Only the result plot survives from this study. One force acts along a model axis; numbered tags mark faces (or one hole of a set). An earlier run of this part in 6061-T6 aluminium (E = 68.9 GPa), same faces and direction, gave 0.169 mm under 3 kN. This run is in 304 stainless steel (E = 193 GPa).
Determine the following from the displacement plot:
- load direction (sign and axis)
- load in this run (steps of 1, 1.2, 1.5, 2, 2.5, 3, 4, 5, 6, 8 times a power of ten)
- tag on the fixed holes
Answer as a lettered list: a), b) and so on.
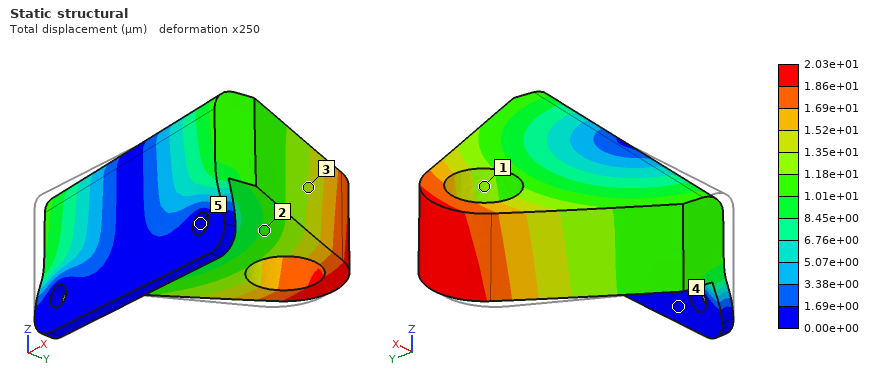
a) +X
b) 1 kN
c) 5
